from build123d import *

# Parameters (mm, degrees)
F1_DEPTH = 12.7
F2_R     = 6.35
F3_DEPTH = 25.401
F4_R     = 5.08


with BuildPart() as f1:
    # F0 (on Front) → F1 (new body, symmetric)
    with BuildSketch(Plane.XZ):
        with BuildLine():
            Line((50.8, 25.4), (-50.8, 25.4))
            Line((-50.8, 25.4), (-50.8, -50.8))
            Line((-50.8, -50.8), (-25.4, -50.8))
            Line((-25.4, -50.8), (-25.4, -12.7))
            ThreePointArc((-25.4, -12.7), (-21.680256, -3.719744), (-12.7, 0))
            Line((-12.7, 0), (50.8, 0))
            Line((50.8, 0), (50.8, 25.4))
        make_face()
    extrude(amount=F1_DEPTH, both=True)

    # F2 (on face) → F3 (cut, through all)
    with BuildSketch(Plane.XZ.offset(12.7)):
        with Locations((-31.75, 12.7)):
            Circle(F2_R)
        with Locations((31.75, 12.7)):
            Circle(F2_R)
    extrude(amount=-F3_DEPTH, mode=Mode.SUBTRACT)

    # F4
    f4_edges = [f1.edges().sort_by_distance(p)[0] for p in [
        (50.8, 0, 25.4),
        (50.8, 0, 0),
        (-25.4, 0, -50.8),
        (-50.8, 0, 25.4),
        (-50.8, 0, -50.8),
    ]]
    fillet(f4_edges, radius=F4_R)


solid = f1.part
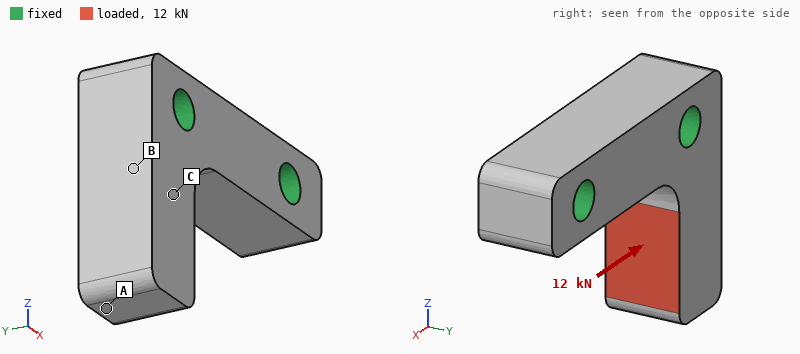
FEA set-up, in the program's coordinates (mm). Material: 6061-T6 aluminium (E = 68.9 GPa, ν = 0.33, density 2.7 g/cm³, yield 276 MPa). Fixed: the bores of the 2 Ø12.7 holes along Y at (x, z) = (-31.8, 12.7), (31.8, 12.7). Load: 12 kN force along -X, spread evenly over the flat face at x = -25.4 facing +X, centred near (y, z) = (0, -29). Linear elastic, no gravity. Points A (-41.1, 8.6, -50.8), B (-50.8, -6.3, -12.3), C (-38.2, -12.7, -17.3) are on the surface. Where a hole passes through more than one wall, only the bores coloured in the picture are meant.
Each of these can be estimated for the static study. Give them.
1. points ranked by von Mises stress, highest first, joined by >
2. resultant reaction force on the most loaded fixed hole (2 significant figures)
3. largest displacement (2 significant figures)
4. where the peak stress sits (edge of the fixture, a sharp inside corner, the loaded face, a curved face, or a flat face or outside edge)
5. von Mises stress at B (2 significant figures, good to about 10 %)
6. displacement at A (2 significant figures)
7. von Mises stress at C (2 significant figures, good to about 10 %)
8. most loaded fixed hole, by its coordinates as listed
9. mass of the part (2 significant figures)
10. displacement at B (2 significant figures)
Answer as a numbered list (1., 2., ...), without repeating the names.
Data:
1. B > C > A
2. 9.6 kN
3. 0.21 mm
4. edge of the fixture
5. 68 MPa
6. 0.20 mm
7. 45 MPa
8. (-31.8, 12.7)
9. 250 g
10. 0.072 mm
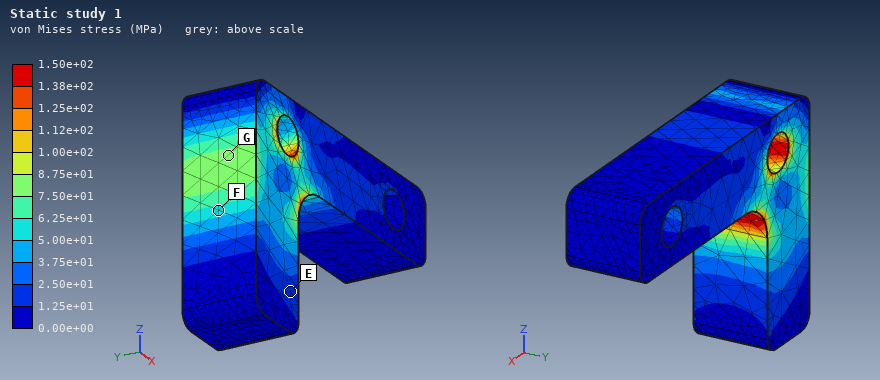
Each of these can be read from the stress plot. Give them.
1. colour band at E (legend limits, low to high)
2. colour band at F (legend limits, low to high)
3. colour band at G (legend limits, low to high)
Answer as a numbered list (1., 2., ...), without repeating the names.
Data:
1. 1.25e+01 to 2.50e+01 MPa
2. 5.00e+01 to 6.25e+01 MPa
3. 7.50e+01 to 8.75e+01 MPa
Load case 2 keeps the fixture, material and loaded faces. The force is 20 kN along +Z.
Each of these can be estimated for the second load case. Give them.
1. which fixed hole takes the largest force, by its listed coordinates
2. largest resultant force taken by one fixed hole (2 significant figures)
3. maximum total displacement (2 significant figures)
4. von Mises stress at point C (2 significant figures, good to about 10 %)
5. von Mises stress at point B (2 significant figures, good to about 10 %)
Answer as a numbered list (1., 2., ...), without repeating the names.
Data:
1. (-31.8, 12.7)
2. 19 kN
3. 0.13 mm
4. 19 MPa
5. 51 MPa
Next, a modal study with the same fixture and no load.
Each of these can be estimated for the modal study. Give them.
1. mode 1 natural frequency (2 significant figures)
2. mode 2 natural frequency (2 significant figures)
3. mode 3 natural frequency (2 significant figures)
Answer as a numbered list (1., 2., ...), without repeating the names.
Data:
1. 5200 Hz
2. 5200 Hz
3. 13 kHz
